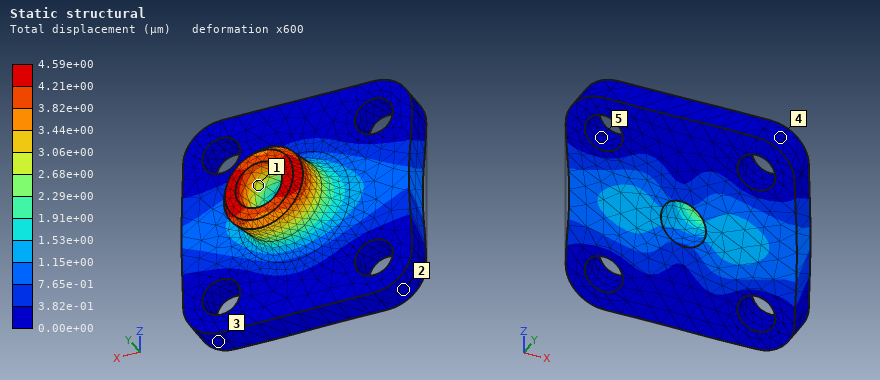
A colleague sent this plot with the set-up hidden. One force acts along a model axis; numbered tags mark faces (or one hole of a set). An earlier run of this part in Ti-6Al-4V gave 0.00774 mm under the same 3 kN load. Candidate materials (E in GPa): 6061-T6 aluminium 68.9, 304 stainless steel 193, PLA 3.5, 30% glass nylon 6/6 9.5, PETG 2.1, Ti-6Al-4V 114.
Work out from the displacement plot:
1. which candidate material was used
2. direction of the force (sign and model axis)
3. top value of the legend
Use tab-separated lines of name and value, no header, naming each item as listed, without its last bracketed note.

which candidate material was used	304 stainless steel
direction of the force	+X
top value of the legend	4.59e+00 µm
